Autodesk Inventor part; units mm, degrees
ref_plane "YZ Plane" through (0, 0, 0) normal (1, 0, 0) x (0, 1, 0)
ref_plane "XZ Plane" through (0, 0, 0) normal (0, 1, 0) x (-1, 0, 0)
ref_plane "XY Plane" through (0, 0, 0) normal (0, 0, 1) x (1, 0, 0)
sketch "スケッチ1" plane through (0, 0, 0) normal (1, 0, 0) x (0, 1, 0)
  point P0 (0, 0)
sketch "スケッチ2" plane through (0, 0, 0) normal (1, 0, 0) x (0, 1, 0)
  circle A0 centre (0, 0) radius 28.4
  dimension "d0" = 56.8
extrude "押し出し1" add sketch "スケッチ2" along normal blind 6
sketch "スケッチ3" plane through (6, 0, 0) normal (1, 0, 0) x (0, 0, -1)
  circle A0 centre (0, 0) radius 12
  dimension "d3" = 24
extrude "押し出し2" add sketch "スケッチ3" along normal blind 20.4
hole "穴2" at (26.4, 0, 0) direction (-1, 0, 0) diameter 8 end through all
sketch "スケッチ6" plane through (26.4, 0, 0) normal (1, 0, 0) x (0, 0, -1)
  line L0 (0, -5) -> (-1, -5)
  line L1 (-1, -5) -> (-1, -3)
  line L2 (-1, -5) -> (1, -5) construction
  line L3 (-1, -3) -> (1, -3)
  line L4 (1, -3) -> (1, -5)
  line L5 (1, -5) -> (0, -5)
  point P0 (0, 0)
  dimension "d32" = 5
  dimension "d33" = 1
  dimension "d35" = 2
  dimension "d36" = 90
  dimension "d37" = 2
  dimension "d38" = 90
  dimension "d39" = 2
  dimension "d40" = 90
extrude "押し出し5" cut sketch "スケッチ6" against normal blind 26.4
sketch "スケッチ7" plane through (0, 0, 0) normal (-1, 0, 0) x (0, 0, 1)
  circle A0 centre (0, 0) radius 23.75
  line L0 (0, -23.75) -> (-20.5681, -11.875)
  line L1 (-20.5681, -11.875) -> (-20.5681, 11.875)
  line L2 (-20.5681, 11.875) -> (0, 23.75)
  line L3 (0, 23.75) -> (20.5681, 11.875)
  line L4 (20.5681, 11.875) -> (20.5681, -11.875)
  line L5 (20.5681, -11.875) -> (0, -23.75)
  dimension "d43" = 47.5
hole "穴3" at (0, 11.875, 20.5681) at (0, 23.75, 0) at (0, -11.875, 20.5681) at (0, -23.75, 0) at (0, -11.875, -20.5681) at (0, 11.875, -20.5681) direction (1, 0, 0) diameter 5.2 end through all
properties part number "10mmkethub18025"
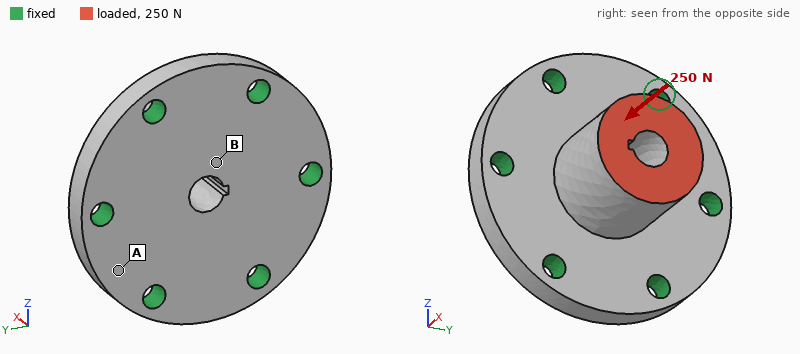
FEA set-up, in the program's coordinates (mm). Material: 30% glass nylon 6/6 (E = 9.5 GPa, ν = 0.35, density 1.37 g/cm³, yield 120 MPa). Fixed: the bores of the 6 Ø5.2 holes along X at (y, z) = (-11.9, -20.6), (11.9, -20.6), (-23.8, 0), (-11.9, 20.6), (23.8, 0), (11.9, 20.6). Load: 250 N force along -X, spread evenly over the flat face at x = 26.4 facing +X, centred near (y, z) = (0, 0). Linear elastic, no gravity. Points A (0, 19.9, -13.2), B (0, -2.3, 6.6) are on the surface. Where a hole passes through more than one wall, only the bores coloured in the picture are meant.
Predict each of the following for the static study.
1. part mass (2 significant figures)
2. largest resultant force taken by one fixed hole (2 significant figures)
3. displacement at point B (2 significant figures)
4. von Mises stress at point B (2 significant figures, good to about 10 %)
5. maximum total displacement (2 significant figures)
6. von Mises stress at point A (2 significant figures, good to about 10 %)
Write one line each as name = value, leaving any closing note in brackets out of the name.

part mass = 31 g
largest resultant force taken by one fixed hole = 45 N
displacement at point B = 5.6 µm
von Mises stress at point B = 1.1 MPa
maximum total displacement = 6.5 µm
von Mises stress at point A = 0.49 MPa
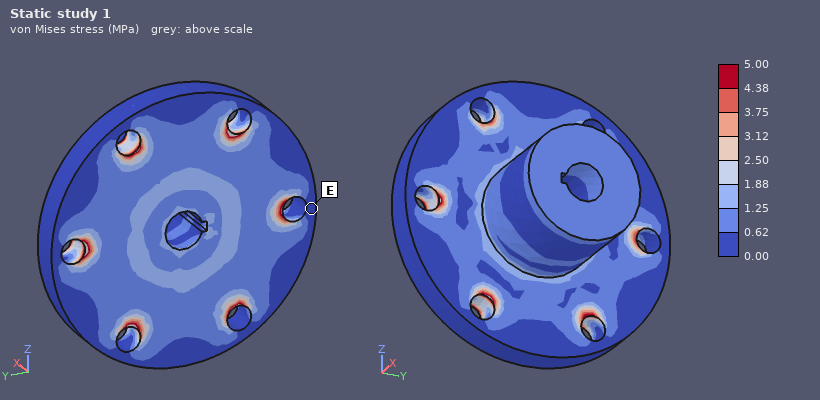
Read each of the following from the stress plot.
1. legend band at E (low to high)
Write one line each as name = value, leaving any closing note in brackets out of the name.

legend band at E = 0.00 to 0.62 MPa
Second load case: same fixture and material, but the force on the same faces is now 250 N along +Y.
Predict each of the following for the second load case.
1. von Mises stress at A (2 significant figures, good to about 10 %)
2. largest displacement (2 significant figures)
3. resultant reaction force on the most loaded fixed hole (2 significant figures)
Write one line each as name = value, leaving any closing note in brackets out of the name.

von Mises stress at A = 1.1 MPa
largest displacement = 30 µm
resultant reaction force on the most loaded fixed hole = 120 N
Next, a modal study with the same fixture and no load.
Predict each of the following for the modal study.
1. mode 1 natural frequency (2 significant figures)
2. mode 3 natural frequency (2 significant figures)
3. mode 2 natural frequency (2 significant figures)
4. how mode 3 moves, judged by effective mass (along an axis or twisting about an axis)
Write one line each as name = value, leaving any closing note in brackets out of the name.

mode 1 natural frequency = 7000 Hz
mode 3 natural frequency = 8300 Hz
mode 2 natural frequency = 7000 Hz
how mode 3 moves, judged by effective mass = along X
